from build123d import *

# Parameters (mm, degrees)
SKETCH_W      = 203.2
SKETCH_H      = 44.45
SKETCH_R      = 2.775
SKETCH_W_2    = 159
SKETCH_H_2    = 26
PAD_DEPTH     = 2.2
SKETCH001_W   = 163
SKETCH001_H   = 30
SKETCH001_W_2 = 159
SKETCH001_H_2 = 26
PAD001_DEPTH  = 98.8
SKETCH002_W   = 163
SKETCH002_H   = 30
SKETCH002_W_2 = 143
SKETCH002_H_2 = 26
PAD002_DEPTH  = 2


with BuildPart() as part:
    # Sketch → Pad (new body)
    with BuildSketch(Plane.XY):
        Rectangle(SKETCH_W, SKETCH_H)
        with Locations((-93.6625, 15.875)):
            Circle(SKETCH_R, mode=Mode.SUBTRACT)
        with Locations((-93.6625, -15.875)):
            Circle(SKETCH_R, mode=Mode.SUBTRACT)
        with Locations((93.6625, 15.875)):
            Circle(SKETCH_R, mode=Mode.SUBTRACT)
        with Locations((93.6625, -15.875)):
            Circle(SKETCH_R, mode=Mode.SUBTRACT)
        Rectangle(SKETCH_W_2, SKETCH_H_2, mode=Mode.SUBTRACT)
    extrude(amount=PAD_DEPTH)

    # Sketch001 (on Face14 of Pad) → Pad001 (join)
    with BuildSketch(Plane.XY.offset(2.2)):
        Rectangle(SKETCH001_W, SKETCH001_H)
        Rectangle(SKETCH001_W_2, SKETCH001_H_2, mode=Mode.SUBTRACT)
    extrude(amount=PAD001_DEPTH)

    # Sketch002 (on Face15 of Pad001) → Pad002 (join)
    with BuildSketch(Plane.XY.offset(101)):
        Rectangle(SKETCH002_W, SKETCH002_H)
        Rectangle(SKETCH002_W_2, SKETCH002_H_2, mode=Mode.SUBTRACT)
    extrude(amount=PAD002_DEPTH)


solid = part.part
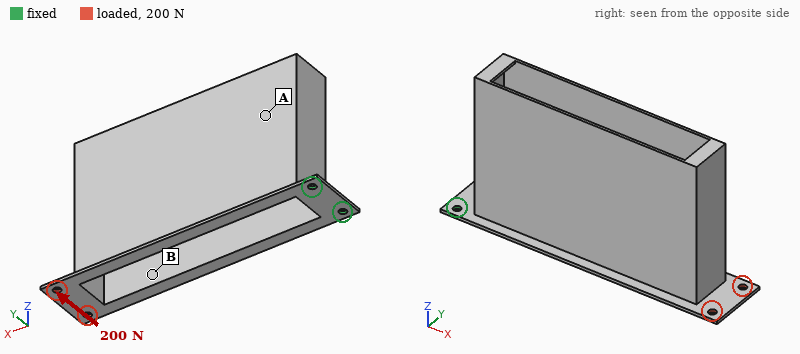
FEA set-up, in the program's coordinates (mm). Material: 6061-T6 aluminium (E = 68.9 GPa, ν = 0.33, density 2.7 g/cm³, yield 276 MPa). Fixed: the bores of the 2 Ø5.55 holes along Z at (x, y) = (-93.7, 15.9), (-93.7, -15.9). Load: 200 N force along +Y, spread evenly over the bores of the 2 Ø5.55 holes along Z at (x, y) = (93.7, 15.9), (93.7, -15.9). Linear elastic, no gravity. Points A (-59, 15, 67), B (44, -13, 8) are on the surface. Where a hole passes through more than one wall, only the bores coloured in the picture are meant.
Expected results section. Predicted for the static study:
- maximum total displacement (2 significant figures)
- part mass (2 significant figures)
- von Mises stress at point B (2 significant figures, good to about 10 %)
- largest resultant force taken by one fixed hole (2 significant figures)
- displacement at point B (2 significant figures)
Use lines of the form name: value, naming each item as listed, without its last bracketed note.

maximum total displacement: 2.5 mm
part mass: 240 g
von Mises stress at point B: 33 MPa
largest resultant force taken by one fixed hole: 1.1 kN
displacement at point B: 1.9 mm
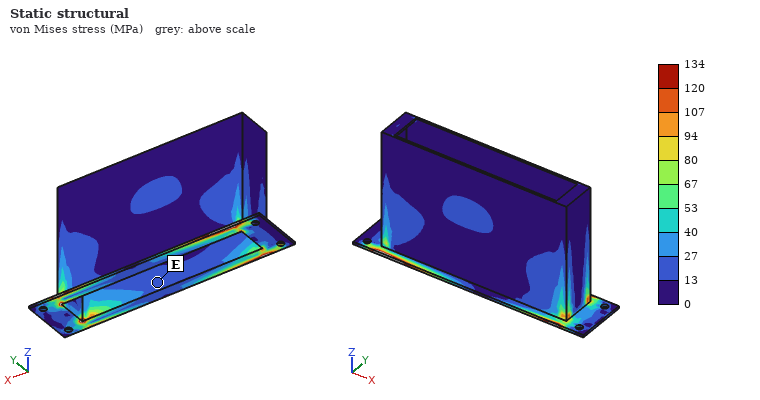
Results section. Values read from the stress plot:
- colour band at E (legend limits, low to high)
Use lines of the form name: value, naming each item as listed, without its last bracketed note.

colour band at E: 13 to 27 MPa
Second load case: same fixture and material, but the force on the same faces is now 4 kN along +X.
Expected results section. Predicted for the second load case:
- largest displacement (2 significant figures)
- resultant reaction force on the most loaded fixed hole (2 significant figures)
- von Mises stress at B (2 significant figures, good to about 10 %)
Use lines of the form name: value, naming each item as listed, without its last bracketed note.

largest displacement: 0.78 mm
resultant reaction force on the most loaded fixed hole: 2.0 kN
von Mises stress at B: 27 MPa
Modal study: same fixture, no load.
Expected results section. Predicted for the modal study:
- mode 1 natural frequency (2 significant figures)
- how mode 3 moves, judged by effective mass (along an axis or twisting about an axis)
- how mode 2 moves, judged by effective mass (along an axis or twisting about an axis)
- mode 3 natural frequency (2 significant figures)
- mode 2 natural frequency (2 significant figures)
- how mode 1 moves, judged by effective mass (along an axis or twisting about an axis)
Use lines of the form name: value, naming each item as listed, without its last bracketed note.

mode 1 natural frequency: 39 Hz
how mode 3 moves, judged by effective mass: twisting about X
how mode 2 moves, judged by effective mass: along Y
mode 3 natural frequency: 290 Hz
mode 2 natural frequency: 140 Hz
how mode 1 moves, judged by effective mass: along Z
